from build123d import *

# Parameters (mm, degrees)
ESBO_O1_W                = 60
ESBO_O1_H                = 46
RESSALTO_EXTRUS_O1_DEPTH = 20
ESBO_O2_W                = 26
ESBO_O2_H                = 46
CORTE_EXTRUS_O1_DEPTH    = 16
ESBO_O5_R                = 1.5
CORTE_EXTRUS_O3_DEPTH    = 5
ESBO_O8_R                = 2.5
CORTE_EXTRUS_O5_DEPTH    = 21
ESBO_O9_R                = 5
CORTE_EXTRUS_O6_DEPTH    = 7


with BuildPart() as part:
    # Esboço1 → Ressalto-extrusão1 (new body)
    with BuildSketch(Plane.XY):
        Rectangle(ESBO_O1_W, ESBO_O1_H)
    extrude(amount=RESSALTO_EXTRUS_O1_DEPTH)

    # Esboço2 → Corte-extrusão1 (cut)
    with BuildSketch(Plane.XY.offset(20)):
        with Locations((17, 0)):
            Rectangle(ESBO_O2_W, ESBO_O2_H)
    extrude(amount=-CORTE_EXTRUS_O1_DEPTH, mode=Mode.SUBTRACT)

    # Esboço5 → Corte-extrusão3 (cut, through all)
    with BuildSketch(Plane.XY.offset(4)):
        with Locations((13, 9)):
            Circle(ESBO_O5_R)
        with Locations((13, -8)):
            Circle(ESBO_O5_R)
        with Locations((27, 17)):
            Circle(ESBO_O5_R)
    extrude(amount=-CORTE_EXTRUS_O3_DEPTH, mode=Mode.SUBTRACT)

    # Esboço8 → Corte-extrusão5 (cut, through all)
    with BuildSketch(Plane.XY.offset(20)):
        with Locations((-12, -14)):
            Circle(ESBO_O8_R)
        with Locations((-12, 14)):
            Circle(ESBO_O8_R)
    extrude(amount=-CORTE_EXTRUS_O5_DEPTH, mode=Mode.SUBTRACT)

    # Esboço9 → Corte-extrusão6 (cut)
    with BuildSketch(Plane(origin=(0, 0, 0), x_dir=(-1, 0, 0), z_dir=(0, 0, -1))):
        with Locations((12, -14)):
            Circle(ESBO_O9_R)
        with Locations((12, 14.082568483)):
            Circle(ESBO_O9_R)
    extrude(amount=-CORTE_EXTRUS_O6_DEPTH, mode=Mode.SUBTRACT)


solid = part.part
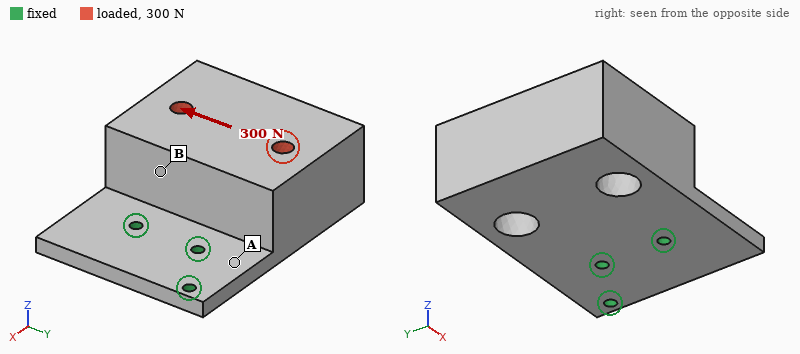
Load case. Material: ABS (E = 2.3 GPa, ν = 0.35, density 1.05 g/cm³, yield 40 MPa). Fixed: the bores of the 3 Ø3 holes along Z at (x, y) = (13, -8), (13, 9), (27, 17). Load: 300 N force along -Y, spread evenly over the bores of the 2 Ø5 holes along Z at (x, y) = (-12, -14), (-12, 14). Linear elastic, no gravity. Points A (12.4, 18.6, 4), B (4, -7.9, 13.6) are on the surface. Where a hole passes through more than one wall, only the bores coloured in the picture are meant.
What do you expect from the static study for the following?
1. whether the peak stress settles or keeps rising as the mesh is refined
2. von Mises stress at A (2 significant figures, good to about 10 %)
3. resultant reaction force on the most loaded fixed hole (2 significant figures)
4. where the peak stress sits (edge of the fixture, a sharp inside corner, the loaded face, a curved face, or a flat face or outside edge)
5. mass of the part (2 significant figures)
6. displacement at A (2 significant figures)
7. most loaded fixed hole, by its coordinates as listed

keeps rising
5.0 MPa
390 N
edge of the fixture
36 g
0.090 mm
(13, -8)
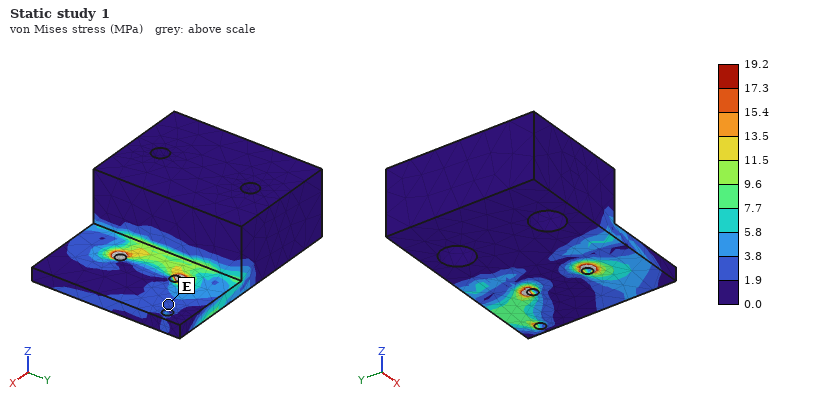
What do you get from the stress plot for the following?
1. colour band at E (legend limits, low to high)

1.9 to 3.8 MPa
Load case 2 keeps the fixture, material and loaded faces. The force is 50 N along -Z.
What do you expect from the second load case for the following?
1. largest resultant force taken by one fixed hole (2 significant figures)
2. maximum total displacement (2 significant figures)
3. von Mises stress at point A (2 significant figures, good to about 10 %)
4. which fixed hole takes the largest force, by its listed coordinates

46 N
0.90 mm
5.5 MPa
(13, 9)
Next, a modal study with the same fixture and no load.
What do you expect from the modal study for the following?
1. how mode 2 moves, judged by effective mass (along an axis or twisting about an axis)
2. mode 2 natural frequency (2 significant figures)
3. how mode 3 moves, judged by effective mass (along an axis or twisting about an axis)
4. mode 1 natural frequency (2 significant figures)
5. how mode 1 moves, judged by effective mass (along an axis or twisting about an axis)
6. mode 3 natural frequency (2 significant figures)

along Y
900 Hz
along Y
240 Hz
along Z
1400 Hz
